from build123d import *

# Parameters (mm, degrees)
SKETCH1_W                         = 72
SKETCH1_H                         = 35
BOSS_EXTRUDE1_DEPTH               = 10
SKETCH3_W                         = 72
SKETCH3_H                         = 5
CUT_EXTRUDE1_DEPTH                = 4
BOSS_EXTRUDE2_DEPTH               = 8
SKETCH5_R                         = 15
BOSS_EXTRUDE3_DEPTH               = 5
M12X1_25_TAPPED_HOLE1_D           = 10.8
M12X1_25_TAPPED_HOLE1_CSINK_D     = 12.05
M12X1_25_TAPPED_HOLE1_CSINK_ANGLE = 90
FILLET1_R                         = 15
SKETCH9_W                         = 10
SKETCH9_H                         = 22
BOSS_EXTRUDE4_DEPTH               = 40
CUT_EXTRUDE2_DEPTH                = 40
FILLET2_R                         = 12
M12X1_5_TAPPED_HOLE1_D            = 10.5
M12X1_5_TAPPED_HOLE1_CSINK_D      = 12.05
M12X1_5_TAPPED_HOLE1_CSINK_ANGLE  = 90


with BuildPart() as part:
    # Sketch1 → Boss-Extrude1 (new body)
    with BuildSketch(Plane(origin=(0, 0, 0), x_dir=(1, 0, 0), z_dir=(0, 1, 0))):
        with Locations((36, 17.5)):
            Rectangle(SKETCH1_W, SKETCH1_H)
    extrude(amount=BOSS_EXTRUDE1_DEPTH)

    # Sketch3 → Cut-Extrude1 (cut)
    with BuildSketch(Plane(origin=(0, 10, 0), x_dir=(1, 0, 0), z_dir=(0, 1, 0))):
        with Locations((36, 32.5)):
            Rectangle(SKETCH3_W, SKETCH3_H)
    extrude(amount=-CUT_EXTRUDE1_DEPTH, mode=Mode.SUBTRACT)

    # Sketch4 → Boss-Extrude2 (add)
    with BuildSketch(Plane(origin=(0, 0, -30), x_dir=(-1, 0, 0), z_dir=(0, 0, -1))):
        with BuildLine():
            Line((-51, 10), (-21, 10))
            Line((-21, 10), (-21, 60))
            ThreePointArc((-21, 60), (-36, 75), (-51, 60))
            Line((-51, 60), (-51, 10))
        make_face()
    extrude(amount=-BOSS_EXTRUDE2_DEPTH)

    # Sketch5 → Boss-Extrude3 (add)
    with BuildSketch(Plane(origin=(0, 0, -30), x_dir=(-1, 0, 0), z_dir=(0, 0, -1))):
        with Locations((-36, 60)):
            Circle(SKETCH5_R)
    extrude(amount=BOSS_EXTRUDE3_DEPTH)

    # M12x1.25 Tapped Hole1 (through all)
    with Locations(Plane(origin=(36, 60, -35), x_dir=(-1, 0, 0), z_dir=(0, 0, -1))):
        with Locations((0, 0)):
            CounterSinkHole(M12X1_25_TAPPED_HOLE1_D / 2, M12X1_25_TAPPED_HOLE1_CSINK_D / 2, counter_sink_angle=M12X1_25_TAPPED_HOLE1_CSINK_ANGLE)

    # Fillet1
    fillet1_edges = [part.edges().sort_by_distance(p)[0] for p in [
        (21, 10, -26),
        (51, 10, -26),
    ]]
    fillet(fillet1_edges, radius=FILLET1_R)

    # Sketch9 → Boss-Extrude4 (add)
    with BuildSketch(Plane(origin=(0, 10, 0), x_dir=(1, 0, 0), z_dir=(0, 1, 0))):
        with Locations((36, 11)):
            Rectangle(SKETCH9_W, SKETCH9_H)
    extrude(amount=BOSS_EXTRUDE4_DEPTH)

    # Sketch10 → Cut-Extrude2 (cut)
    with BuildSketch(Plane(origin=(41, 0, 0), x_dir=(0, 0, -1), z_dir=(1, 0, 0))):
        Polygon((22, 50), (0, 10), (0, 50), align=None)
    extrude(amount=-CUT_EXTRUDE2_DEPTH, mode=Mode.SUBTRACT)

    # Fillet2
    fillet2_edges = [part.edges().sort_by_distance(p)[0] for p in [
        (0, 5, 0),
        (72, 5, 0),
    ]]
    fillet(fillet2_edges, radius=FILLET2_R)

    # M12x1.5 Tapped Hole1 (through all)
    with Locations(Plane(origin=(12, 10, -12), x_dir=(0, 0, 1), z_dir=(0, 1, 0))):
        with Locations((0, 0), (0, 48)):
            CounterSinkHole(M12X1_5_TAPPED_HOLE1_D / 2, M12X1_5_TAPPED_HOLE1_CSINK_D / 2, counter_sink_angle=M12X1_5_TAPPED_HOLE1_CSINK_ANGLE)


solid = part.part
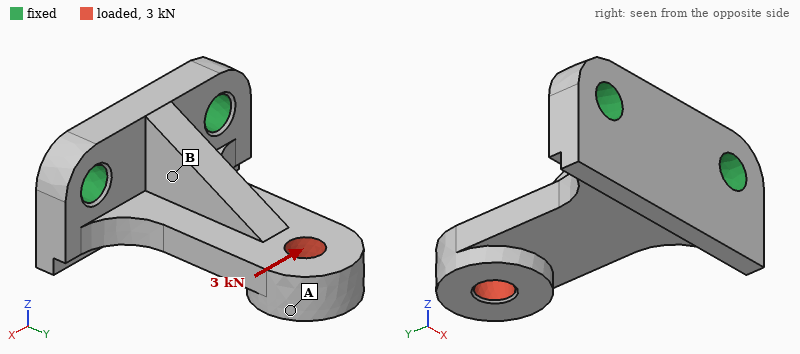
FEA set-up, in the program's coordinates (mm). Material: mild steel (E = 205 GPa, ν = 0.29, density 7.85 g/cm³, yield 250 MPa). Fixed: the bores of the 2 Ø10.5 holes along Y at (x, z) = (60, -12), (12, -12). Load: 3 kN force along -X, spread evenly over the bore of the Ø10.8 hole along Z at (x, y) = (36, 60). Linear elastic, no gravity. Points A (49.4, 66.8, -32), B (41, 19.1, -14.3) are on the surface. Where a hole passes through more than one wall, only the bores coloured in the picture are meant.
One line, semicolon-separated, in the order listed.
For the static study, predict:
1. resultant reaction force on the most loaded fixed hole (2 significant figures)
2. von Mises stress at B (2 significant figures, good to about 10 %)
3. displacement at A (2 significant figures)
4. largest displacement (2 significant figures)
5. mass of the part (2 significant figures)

4.2 kN; 29 MPa; 62 µm; 70 µm; 340 g
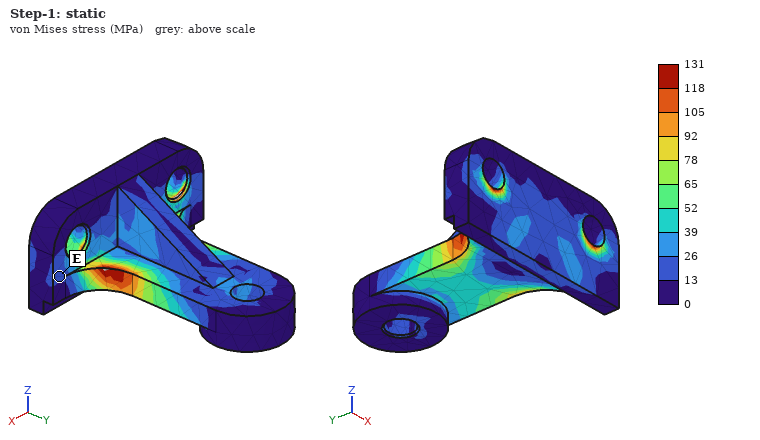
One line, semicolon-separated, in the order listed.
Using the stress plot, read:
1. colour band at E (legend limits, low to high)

13 to 26 MPa
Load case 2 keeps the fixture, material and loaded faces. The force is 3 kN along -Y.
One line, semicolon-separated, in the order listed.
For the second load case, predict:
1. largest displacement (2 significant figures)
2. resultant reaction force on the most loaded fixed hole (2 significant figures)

39 µm; 1.5 kN
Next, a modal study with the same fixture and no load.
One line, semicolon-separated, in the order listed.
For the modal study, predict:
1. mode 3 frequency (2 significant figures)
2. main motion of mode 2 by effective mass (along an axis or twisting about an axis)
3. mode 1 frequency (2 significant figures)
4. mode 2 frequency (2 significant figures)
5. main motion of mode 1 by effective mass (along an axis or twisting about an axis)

7800 Hz; along X; 2500 Hz; 4300 Hz; along Z
